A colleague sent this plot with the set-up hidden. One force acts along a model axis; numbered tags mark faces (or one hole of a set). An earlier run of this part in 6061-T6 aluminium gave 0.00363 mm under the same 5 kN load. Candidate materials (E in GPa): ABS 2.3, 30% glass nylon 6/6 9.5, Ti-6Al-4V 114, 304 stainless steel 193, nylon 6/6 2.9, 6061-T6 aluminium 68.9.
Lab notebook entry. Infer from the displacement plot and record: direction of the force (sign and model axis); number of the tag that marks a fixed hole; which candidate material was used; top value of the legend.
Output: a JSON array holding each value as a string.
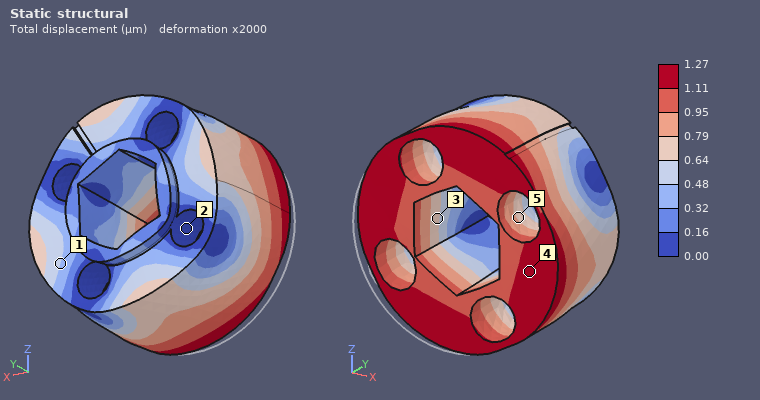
["+Y", "2", "304 stainless steel", "1.27 µm"]
